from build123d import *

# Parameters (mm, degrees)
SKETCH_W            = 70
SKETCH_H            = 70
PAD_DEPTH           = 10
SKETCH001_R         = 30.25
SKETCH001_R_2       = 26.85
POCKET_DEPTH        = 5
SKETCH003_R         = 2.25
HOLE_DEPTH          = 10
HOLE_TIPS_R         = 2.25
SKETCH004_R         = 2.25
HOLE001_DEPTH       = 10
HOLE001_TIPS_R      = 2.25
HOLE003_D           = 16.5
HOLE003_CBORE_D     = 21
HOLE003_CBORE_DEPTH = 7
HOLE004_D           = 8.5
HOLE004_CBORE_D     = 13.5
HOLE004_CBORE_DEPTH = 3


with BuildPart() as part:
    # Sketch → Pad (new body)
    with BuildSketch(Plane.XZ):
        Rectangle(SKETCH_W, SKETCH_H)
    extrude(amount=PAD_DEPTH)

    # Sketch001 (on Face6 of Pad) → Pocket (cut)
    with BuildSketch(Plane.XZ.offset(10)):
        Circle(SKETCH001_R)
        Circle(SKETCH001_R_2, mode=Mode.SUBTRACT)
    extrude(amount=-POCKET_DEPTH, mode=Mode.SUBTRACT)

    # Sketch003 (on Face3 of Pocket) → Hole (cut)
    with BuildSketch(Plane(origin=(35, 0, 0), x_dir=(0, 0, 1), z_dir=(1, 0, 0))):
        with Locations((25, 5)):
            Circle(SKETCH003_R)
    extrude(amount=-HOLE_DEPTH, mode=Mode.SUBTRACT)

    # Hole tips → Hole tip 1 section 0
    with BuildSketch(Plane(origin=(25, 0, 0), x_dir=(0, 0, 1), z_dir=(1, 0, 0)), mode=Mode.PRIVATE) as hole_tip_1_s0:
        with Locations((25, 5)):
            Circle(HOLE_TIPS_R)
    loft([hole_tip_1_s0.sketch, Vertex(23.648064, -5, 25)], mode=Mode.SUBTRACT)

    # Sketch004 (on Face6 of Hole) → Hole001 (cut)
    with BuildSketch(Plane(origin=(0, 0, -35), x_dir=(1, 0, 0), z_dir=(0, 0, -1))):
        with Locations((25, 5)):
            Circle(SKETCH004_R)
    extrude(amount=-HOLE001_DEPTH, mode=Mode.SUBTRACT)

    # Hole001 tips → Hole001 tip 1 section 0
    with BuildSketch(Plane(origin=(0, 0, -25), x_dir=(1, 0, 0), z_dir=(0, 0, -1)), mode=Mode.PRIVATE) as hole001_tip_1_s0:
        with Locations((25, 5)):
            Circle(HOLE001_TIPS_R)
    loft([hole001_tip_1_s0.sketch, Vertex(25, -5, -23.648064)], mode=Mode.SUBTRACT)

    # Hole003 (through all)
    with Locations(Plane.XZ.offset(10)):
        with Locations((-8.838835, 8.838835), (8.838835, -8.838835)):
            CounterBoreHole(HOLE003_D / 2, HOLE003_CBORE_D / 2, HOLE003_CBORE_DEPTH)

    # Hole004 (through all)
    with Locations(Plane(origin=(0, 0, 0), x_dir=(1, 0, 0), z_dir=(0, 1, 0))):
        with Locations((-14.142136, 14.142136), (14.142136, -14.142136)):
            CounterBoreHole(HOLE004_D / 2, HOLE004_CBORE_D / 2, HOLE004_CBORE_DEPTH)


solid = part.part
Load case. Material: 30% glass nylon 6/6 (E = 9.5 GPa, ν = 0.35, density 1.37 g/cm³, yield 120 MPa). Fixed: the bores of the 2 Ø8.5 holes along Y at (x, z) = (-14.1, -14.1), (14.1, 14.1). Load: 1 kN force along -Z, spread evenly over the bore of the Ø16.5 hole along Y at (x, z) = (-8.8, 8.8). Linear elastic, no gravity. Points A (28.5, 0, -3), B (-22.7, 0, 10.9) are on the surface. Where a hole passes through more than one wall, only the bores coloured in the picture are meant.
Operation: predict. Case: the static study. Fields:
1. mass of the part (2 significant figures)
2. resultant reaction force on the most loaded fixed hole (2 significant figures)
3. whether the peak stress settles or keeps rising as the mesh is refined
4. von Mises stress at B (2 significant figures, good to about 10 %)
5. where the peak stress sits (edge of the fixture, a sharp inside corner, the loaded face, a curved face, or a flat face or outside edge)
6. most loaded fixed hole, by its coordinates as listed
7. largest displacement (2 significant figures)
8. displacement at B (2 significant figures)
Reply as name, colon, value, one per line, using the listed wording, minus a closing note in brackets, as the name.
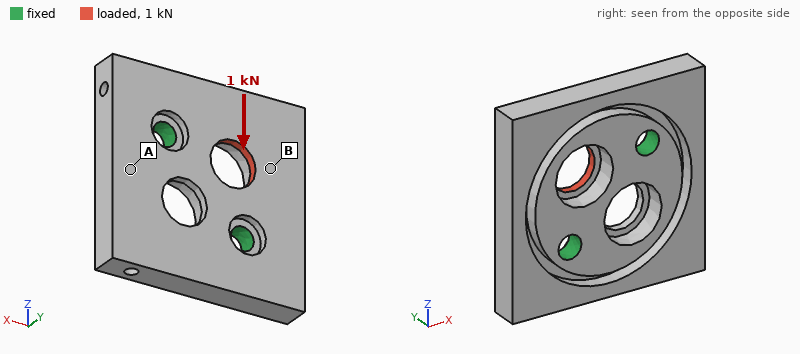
mass of the part: 52 g
resultant reaction force on the most loaded fixed hole: 670 N
whether the peak stress settles or keeps rising as the mesh is refined: keeps rising
von Mises stress at B: 2.8 MPa
where the peak stress sits: edge of the fixture
most loaded fixed hole, by its coordinates as listed: (-14.1, -14.1)
largest displacement: 67 µm
displacement at B: 27 µm
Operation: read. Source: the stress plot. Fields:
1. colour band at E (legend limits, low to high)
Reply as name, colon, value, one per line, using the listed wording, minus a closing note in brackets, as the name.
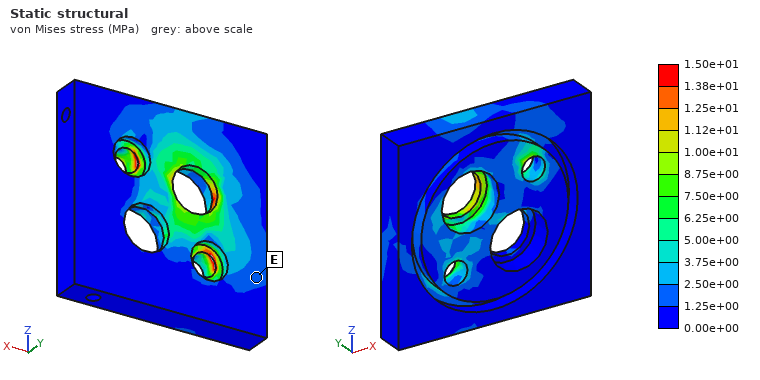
colour band at E: 1.25e+00 to 2.50e+00 MPa
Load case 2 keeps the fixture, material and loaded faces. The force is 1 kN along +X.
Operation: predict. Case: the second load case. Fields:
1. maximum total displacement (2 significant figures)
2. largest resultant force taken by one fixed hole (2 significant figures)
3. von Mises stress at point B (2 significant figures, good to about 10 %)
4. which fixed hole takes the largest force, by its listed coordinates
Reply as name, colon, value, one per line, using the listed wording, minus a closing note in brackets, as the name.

maximum total displacement: 67 µm
largest resultant force taken by one fixed hole: 670 N
von Mises stress at point B: 4.5 MPa
which fixed hole takes the largest force, by its listed coordinates: (14.1, 14.1)
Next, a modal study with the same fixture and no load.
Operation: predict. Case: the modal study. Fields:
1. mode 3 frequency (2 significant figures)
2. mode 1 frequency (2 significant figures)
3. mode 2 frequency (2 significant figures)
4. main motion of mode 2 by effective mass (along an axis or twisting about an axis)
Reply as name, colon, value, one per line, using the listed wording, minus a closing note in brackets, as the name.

mode 3 frequency: 4000 Hz
mode 1 frequency: 2000 Hz
mode 2 frequency: 2300 Hz
main motion of mode 2 by effective mass: along Y
